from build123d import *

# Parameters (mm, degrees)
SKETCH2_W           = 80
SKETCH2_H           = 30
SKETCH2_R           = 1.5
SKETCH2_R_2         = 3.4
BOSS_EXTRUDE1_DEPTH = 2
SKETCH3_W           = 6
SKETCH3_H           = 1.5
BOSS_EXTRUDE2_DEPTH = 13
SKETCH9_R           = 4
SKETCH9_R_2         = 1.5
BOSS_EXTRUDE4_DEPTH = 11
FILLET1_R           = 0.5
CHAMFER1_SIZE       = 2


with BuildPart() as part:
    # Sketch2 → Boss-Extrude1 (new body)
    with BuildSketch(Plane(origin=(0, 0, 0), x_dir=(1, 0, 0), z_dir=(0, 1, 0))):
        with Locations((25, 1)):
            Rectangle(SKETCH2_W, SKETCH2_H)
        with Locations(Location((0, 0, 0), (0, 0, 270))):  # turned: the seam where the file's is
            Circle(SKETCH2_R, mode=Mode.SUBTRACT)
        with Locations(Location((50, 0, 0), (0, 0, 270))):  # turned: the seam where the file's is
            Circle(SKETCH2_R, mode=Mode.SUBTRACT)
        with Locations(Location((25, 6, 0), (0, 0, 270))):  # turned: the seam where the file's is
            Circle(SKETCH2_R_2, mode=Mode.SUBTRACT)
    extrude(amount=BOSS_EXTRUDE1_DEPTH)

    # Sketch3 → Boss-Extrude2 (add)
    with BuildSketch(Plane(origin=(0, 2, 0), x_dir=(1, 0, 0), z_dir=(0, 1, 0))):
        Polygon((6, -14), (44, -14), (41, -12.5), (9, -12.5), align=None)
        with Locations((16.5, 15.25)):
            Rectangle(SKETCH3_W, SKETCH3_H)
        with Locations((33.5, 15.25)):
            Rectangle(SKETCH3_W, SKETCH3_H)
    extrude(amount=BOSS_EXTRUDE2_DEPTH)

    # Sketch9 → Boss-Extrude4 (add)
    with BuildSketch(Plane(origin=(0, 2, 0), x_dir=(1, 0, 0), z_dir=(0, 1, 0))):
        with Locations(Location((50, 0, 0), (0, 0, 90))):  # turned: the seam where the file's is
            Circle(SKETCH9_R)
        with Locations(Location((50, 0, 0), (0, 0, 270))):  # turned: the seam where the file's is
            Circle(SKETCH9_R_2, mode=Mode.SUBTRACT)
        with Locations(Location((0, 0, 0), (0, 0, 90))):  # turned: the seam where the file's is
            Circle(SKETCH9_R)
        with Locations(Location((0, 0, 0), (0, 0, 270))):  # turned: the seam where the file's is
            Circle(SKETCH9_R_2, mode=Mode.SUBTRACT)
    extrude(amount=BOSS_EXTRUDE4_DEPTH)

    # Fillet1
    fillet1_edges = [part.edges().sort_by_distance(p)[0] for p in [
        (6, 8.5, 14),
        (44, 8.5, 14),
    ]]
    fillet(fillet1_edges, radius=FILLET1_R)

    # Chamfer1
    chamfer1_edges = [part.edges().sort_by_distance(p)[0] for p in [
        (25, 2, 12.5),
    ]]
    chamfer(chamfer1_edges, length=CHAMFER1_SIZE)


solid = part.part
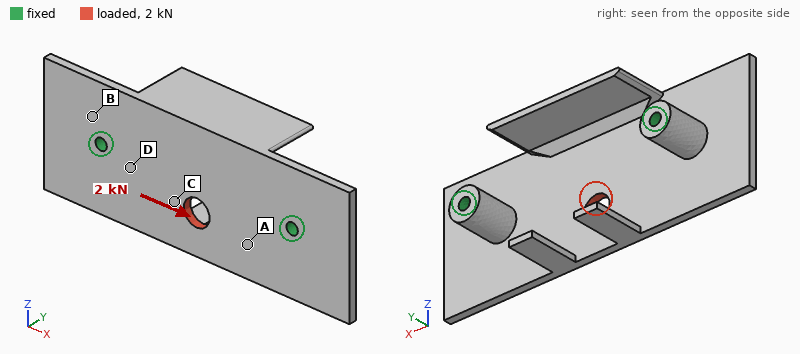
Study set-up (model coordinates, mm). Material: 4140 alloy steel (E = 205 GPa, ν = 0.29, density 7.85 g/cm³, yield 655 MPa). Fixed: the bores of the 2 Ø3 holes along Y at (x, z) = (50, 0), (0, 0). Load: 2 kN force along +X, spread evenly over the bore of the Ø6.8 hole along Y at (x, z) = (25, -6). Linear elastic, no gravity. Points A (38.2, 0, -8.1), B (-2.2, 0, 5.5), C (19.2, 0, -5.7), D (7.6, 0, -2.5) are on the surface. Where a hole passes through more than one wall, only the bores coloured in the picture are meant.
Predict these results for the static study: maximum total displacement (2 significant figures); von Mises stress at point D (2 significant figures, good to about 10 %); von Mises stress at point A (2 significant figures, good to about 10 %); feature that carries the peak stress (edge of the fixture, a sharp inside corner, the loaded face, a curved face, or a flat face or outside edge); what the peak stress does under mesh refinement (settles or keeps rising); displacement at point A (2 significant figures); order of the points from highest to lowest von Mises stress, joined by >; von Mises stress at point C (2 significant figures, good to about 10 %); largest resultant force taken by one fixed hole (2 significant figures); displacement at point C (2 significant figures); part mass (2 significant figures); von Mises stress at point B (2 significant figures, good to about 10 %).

4.7 µm
33 MPa
26 MPa
edge of the fixture
keeps rising
2.5 µm
C > D > A > B
46 MPa
1.0 kN
3.4 µm
52 g
12 MPa
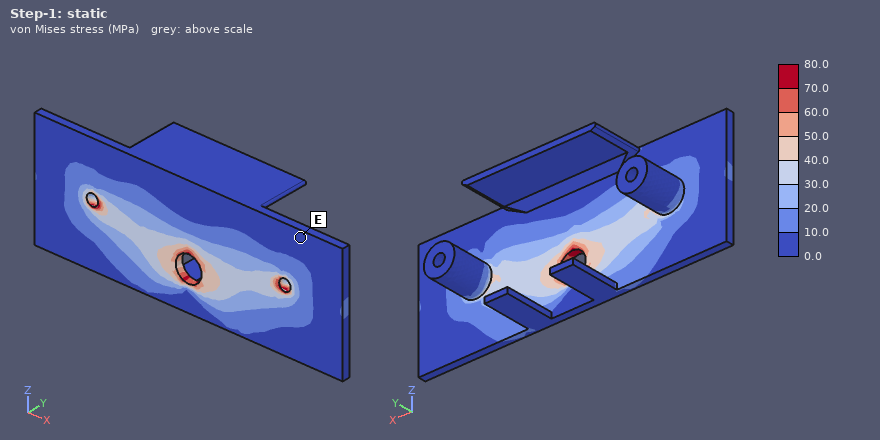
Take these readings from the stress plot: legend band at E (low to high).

0.0 to 10.0 MPa
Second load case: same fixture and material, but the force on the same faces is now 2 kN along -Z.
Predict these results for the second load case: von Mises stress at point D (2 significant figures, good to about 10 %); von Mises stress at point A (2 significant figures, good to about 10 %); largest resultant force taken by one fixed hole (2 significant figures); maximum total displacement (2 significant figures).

38 MPa
33 MPa
1.0 kN
11 µm
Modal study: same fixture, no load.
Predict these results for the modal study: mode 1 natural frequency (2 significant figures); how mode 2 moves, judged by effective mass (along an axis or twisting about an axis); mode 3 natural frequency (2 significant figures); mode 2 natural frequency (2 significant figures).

3200 Hz
along Y
5400 Hz
4000 Hz
